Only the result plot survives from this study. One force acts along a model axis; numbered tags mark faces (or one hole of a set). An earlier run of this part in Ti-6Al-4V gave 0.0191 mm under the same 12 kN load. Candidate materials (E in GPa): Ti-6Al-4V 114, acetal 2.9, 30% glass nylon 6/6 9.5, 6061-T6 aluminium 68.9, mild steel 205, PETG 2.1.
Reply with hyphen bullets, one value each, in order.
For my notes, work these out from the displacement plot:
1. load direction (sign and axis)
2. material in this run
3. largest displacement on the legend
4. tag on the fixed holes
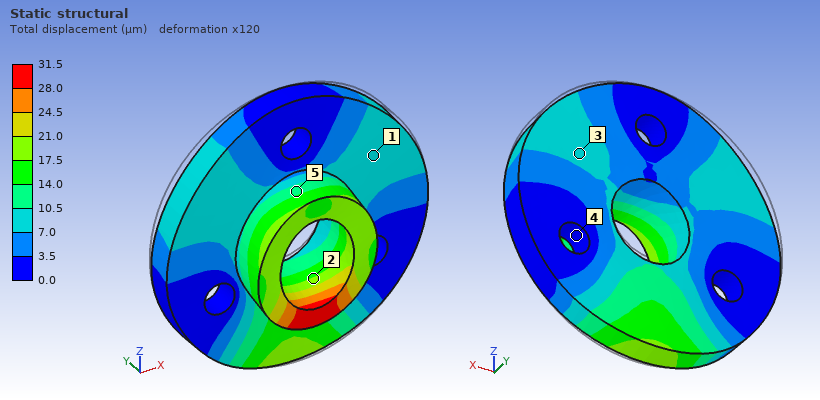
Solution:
- -Z
- 6061-T6 aluminium
- 31.5 µm
- 4
